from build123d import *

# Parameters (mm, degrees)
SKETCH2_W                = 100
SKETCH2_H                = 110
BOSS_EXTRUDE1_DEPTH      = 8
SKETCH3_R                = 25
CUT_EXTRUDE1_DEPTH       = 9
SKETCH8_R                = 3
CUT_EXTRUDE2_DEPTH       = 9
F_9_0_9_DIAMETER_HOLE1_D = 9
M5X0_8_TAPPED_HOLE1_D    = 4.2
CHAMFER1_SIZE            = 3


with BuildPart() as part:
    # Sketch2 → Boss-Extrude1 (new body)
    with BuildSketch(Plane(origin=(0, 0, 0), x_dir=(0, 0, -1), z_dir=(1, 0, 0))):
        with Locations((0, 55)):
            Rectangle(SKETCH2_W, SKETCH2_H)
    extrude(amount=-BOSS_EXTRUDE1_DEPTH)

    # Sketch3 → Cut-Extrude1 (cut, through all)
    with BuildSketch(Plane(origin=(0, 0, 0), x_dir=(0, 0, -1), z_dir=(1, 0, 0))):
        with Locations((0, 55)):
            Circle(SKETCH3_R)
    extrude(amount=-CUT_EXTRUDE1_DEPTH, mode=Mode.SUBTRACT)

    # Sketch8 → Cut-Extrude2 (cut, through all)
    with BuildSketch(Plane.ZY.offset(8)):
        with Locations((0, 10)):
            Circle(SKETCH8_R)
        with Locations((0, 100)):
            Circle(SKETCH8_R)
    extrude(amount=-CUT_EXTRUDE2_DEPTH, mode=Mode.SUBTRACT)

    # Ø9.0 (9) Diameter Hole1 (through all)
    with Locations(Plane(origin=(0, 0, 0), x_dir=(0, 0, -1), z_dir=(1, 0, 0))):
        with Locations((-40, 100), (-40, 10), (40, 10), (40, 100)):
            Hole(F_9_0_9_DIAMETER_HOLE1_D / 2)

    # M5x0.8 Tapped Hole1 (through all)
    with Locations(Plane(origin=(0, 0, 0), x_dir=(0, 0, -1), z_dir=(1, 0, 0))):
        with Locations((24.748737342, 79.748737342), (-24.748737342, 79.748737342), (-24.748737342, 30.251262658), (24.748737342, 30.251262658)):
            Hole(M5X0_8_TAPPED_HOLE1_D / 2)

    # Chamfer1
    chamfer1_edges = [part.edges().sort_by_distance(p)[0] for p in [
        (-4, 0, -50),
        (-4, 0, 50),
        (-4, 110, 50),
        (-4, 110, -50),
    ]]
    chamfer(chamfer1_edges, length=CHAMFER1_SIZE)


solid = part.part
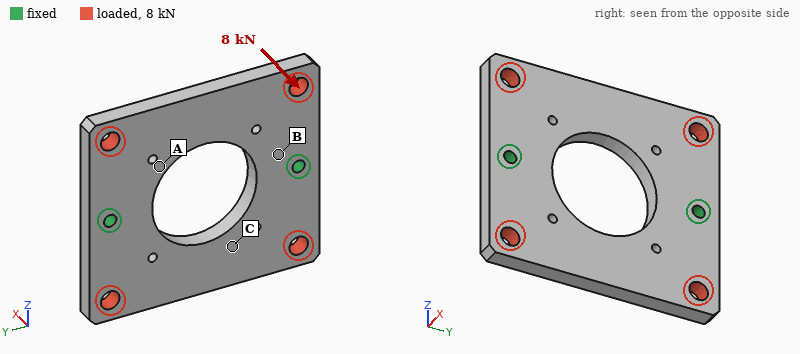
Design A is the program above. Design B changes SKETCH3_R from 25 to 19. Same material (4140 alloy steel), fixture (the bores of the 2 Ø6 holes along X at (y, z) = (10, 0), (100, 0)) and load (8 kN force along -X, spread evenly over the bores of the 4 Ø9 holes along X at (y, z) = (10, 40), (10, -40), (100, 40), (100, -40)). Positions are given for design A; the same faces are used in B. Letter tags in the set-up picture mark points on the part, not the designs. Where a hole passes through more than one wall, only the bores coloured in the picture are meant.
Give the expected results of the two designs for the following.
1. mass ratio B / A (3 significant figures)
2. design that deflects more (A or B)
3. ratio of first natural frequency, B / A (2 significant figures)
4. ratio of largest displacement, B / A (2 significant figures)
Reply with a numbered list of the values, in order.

1. 1.10
2. A
3. 1.0
4. 0.87
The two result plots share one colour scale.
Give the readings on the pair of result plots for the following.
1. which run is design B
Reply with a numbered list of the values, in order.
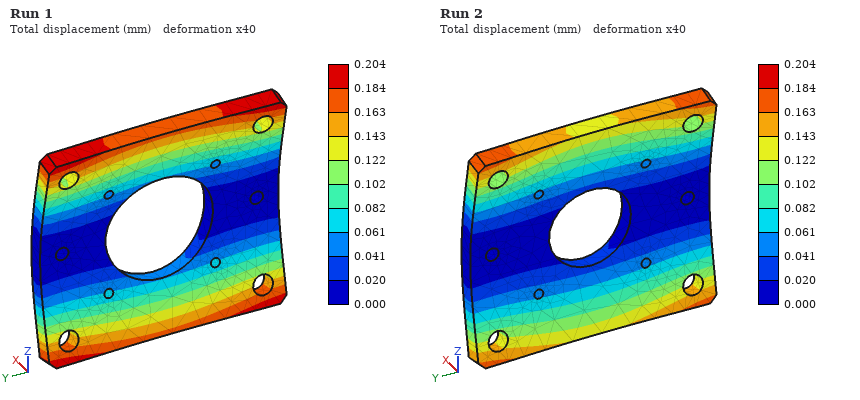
1. Run 2
